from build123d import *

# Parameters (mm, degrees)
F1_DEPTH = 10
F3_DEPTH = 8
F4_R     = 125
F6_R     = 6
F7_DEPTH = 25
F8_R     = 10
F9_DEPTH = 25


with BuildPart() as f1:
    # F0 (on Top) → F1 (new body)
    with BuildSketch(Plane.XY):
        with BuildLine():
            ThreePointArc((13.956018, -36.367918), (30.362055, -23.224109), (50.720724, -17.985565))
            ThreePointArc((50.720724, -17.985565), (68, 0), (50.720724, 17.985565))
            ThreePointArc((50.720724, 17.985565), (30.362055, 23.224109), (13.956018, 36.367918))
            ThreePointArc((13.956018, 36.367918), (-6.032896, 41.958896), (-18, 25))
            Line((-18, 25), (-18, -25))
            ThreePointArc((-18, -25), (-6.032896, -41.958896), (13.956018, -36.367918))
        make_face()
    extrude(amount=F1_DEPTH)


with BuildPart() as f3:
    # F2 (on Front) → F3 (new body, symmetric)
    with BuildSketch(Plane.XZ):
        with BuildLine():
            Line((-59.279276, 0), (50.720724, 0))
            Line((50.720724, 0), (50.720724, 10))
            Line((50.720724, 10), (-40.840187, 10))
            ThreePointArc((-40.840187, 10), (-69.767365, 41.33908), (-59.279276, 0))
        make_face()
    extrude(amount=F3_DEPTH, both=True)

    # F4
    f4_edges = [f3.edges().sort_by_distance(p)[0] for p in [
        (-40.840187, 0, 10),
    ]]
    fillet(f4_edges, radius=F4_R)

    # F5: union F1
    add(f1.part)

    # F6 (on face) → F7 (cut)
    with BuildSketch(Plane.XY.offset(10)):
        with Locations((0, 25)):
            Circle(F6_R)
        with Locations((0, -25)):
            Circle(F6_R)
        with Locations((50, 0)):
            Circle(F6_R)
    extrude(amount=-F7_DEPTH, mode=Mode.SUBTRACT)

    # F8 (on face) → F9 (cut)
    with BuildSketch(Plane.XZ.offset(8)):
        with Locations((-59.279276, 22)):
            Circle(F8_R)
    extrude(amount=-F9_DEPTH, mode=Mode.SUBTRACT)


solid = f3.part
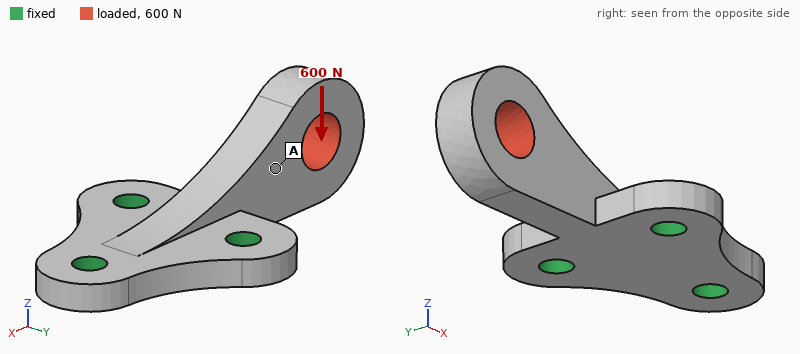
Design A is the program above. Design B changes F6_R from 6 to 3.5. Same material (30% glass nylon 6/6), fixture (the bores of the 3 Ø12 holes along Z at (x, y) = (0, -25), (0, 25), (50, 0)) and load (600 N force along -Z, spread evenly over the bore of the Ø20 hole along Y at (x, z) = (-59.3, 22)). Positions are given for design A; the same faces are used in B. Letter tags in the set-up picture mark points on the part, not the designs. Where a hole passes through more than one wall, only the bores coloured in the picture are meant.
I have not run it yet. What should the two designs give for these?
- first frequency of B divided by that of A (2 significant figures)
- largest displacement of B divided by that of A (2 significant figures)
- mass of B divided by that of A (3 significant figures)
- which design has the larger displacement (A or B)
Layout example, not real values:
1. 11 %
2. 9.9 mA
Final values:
1. 0.93
2. 1.1
3. 1.03
4. B
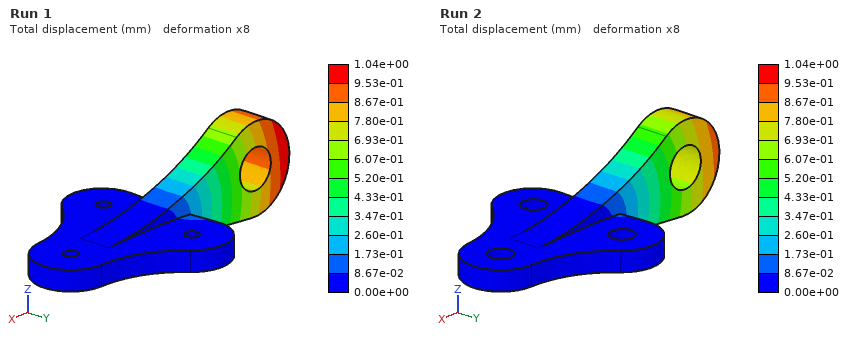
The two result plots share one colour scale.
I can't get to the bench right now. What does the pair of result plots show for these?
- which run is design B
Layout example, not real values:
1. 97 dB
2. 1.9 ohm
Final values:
1. Run 1
